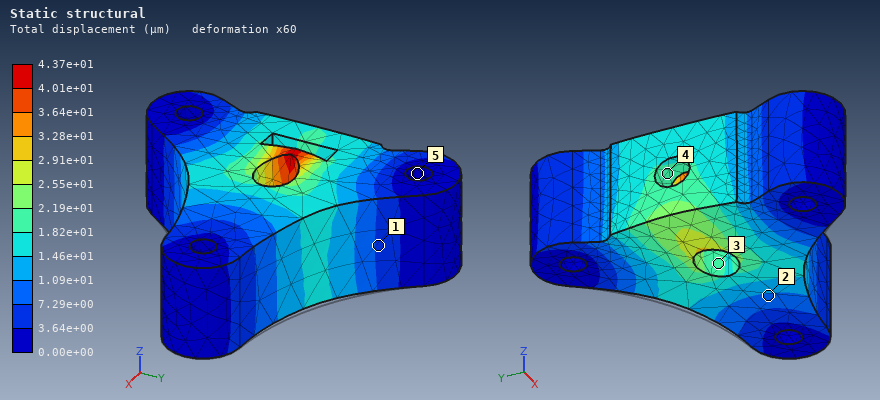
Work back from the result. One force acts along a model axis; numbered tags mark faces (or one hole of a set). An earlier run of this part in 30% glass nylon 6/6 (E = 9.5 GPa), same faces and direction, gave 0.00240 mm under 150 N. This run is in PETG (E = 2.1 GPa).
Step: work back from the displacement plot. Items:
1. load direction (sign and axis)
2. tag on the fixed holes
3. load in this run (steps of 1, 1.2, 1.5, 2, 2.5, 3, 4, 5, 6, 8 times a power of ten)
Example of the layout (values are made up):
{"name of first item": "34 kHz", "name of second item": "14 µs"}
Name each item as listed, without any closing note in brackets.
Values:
{"load direction": "-X", "tag on the fixed holes": "5", "load in this run": "600 N"}
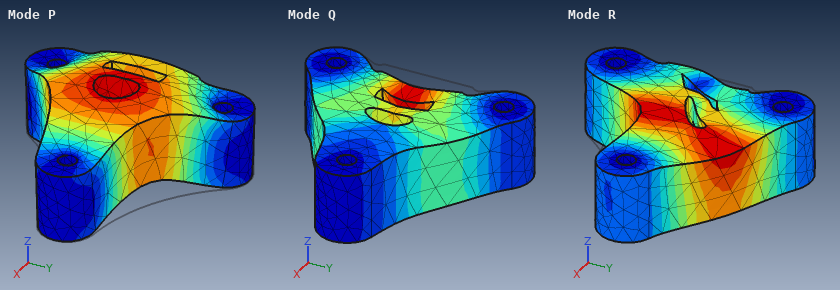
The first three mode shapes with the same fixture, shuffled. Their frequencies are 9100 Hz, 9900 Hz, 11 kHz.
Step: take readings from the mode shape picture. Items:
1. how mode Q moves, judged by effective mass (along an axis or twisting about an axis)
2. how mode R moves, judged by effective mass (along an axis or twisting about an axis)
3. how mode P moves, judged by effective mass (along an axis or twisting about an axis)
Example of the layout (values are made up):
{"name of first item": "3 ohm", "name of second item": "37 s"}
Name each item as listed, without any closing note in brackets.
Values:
{"how mode Q moves, judged by effective mass": "along X", "how mode R moves, judged by effective mass": "along Y", "how mode P moves, judged by effective mass": "along Z"}
